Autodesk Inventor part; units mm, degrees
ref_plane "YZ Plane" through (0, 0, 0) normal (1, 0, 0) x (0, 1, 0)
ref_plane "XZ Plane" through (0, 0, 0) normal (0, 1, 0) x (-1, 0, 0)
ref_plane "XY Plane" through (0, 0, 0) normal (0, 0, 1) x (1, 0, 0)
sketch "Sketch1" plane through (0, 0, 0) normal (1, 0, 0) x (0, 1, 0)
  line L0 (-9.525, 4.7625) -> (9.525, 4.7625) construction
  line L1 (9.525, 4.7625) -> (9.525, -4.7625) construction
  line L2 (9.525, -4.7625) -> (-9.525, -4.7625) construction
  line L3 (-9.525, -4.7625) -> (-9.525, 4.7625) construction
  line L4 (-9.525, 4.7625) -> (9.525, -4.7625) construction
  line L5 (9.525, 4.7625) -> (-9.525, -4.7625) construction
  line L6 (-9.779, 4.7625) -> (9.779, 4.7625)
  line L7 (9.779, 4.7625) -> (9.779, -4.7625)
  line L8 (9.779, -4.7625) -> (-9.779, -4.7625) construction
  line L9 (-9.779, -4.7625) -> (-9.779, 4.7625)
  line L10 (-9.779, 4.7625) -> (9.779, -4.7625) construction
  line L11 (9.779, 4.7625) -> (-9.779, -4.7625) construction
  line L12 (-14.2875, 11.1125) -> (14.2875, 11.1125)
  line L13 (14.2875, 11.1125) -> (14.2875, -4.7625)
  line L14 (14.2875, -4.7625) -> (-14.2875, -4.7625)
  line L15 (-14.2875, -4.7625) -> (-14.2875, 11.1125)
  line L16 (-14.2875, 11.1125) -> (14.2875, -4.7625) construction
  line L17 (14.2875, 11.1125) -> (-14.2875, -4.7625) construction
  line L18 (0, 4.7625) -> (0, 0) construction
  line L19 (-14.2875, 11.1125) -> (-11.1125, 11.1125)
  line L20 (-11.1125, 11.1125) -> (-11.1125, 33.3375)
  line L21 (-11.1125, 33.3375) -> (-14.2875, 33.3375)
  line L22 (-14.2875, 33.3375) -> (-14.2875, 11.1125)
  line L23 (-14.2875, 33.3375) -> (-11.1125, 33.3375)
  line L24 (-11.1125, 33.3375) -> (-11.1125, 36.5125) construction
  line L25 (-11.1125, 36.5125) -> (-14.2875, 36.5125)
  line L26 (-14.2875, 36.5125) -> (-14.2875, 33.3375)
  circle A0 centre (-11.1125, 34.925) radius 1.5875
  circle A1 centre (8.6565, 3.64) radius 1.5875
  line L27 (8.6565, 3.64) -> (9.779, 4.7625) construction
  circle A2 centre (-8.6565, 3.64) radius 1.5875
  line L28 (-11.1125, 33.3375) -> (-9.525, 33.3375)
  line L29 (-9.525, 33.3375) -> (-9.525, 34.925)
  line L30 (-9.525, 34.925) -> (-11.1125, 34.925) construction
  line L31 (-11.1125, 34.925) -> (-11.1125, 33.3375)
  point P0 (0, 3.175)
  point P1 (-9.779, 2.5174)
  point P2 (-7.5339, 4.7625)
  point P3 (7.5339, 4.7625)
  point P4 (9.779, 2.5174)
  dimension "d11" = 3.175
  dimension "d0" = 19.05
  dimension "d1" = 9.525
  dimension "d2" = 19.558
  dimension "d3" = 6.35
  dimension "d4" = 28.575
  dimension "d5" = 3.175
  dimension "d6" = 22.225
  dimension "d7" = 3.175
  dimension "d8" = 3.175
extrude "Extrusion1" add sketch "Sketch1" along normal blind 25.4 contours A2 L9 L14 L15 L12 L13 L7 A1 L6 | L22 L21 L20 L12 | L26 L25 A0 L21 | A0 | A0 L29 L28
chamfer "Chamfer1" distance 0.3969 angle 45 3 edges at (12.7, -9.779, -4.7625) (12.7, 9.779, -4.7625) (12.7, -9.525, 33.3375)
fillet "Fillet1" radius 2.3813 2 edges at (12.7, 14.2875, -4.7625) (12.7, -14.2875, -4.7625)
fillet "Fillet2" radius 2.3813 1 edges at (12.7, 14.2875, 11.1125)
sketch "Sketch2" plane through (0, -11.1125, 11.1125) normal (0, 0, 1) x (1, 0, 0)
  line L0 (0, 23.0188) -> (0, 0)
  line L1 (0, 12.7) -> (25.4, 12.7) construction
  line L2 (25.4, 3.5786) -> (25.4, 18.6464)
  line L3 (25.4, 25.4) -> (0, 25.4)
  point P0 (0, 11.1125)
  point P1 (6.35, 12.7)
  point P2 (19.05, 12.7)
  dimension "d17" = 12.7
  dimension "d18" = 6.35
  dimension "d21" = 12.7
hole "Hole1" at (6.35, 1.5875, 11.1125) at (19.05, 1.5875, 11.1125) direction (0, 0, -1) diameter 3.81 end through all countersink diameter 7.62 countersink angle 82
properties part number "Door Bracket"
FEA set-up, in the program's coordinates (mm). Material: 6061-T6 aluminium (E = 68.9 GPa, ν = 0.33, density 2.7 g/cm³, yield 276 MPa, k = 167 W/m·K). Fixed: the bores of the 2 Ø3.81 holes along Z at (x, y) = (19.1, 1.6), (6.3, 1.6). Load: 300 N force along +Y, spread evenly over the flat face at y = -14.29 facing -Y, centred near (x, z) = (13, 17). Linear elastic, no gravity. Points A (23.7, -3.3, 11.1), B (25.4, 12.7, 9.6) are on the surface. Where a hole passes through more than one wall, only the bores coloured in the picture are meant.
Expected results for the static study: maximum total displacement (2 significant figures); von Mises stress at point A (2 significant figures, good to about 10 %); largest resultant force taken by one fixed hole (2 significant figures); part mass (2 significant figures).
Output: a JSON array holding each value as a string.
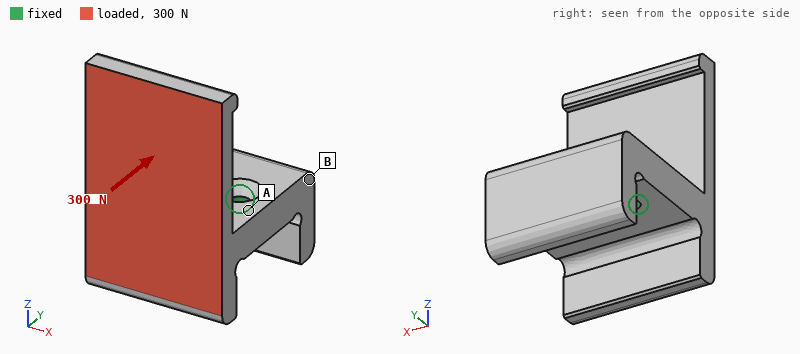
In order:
["0.14 mm", "17 MPa", "150 N", "23 g"]
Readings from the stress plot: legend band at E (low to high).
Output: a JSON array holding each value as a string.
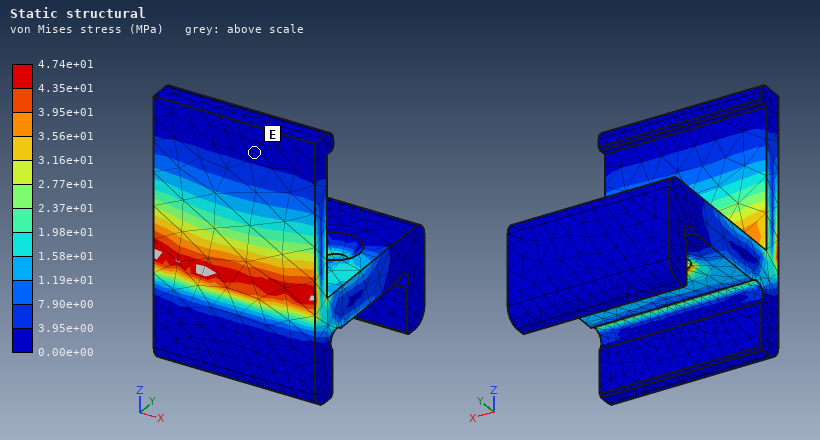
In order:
["0.00e+00 to 3.95e+00 MPa"]
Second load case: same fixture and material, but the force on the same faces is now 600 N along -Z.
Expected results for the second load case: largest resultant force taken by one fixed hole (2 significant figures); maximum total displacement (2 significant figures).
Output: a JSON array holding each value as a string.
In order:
["300 N", "0.12 mm"]
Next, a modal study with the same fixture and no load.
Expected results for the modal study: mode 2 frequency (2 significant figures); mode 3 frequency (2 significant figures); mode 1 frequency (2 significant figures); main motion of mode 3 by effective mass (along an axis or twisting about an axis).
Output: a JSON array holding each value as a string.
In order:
["6300 Hz", "7700 Hz", "2800 Hz", "along Z"]
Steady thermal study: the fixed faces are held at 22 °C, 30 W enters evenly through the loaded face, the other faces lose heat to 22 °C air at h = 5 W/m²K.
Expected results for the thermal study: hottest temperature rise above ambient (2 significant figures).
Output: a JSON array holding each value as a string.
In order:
["36 K"]
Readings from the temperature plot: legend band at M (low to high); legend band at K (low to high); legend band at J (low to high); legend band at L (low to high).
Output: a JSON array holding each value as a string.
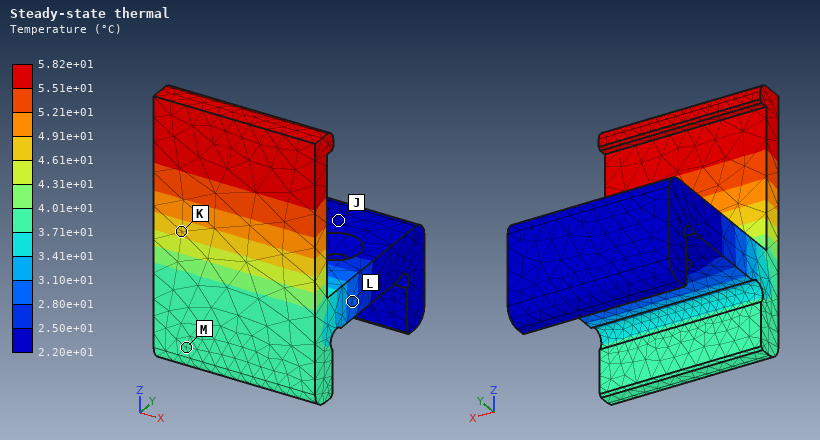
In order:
["3.71e+01 to 4.01e+01 °C", "4.61e+01 to 4.91e+01 °C", "2.20e+01 to 2.50e+01 °C", "2.80e+01 to 3.10e+01 °C"]
